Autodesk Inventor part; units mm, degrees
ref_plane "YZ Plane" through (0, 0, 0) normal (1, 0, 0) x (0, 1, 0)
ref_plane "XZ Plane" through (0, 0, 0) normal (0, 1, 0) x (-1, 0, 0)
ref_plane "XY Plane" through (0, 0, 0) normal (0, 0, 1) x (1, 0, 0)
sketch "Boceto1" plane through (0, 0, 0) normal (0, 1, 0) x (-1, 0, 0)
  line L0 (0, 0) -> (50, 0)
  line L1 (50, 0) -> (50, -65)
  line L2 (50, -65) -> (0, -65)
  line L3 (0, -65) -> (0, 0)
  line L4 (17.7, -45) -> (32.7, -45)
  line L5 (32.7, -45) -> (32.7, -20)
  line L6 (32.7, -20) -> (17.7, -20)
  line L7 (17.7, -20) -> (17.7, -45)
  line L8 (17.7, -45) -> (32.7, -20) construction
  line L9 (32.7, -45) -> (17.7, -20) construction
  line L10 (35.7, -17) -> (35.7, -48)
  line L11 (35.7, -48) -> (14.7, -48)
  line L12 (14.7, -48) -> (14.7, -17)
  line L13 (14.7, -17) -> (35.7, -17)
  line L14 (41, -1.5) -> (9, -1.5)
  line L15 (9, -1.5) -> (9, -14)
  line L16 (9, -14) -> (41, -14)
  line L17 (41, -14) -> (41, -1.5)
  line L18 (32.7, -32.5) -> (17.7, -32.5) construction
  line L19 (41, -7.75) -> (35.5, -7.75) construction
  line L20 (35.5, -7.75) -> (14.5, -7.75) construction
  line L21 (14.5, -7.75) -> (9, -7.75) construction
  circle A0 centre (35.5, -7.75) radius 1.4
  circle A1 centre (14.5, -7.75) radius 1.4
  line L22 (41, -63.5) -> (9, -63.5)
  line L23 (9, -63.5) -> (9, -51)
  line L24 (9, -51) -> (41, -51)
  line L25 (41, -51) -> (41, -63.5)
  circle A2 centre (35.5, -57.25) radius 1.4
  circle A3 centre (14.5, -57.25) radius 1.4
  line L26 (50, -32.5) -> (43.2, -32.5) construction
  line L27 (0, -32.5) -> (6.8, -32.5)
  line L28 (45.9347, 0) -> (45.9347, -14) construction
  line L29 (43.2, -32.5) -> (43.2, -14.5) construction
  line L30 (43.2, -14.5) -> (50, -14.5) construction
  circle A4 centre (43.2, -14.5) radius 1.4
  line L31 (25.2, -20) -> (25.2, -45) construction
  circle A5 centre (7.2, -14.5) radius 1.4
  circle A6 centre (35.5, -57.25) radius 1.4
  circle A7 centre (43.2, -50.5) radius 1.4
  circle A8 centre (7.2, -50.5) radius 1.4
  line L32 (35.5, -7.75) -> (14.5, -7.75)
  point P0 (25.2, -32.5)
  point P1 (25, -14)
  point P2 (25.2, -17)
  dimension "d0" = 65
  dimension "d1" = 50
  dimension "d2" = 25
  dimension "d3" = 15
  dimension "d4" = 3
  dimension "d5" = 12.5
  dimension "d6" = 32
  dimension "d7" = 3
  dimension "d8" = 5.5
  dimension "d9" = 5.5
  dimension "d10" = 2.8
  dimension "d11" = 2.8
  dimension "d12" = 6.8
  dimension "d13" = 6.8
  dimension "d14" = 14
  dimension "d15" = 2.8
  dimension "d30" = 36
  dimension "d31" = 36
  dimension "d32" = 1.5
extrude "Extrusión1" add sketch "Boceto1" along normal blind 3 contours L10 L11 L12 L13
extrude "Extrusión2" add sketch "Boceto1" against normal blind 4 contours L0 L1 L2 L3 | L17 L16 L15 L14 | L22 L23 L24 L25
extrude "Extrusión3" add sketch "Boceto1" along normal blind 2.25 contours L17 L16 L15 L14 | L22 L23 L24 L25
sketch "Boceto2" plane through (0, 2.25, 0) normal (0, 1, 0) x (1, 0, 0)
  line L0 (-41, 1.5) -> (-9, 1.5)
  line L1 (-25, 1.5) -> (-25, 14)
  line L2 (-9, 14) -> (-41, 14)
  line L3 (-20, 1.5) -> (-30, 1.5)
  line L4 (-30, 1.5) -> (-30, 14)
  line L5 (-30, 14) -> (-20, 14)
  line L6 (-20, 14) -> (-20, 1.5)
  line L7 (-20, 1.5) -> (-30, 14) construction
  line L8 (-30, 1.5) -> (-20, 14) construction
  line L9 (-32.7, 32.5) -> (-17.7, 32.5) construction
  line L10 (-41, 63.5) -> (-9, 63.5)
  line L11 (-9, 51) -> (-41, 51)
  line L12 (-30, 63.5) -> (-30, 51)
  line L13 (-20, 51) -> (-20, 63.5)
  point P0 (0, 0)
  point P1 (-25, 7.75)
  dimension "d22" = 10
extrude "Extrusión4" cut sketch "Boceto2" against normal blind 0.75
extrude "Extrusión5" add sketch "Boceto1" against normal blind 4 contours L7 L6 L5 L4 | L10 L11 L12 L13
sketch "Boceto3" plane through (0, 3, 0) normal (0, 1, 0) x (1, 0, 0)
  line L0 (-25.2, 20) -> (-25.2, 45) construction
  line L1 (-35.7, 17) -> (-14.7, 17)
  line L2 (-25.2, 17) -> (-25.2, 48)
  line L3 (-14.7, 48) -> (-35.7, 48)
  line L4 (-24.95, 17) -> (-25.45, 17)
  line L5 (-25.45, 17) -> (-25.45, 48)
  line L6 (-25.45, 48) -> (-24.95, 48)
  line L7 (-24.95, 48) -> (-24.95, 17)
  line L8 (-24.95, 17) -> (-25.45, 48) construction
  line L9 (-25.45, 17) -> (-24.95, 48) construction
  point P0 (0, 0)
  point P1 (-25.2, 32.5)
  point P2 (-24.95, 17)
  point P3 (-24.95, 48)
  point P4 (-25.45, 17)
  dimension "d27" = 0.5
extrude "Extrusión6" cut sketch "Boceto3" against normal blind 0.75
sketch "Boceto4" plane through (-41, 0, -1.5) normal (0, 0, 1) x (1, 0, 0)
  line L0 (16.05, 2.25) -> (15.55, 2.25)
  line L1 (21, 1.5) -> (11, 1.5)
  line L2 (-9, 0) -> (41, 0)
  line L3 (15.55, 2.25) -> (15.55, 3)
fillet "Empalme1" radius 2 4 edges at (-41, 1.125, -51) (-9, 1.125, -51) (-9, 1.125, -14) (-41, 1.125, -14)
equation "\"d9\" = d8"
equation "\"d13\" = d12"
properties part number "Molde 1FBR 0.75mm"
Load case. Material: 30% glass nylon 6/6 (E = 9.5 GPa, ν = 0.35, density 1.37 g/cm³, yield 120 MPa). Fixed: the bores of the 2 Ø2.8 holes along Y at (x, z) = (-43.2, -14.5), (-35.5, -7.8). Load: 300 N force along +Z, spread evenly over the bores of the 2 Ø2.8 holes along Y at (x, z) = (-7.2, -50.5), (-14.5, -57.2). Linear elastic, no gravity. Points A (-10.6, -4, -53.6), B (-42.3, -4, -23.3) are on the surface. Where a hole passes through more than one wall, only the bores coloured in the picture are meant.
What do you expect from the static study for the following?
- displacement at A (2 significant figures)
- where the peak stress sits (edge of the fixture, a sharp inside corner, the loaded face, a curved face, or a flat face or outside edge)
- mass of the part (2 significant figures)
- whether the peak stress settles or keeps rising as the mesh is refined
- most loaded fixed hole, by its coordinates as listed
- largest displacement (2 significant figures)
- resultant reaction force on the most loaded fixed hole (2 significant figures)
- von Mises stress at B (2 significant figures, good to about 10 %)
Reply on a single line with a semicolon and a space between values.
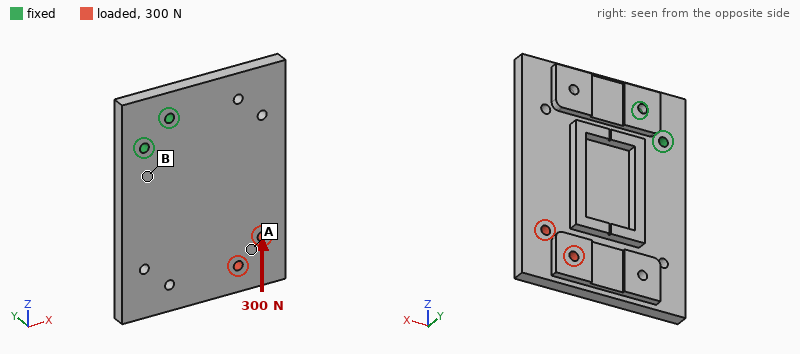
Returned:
0.15 mm; edge of the fixture; 21 g; keeps rising; (-35.5, -7.8); 0.20 mm; 790 N; 4.6 MPa
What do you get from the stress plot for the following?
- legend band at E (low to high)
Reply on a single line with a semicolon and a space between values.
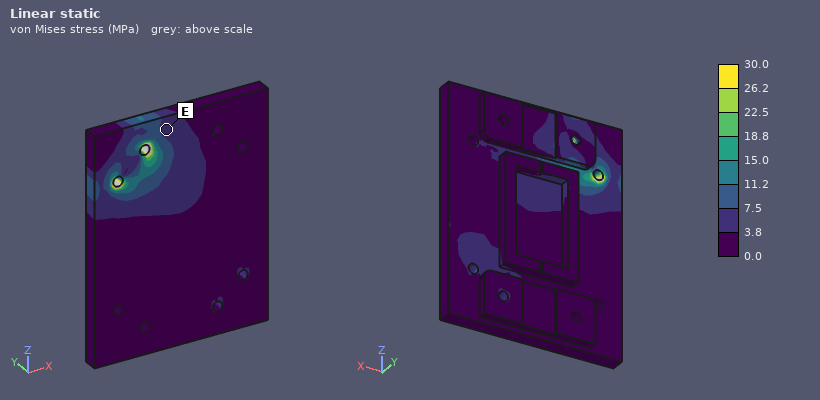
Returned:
3.8 to 7.5 MPa
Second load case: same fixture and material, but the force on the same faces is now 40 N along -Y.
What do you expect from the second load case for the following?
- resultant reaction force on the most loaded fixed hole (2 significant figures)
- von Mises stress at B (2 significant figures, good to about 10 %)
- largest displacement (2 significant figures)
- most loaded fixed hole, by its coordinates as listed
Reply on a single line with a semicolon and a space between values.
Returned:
36 N; 12 MPa; 0.92 mm; (-43.2, -14.5)
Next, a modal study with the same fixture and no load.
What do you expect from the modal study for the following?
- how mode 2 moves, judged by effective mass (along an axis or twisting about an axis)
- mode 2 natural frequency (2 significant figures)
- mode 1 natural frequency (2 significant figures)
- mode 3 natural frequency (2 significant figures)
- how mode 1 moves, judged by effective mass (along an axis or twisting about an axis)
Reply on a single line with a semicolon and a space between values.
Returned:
twisting about Z; 1200 Hz; 490 Hz; 1700 Hz; along Y
